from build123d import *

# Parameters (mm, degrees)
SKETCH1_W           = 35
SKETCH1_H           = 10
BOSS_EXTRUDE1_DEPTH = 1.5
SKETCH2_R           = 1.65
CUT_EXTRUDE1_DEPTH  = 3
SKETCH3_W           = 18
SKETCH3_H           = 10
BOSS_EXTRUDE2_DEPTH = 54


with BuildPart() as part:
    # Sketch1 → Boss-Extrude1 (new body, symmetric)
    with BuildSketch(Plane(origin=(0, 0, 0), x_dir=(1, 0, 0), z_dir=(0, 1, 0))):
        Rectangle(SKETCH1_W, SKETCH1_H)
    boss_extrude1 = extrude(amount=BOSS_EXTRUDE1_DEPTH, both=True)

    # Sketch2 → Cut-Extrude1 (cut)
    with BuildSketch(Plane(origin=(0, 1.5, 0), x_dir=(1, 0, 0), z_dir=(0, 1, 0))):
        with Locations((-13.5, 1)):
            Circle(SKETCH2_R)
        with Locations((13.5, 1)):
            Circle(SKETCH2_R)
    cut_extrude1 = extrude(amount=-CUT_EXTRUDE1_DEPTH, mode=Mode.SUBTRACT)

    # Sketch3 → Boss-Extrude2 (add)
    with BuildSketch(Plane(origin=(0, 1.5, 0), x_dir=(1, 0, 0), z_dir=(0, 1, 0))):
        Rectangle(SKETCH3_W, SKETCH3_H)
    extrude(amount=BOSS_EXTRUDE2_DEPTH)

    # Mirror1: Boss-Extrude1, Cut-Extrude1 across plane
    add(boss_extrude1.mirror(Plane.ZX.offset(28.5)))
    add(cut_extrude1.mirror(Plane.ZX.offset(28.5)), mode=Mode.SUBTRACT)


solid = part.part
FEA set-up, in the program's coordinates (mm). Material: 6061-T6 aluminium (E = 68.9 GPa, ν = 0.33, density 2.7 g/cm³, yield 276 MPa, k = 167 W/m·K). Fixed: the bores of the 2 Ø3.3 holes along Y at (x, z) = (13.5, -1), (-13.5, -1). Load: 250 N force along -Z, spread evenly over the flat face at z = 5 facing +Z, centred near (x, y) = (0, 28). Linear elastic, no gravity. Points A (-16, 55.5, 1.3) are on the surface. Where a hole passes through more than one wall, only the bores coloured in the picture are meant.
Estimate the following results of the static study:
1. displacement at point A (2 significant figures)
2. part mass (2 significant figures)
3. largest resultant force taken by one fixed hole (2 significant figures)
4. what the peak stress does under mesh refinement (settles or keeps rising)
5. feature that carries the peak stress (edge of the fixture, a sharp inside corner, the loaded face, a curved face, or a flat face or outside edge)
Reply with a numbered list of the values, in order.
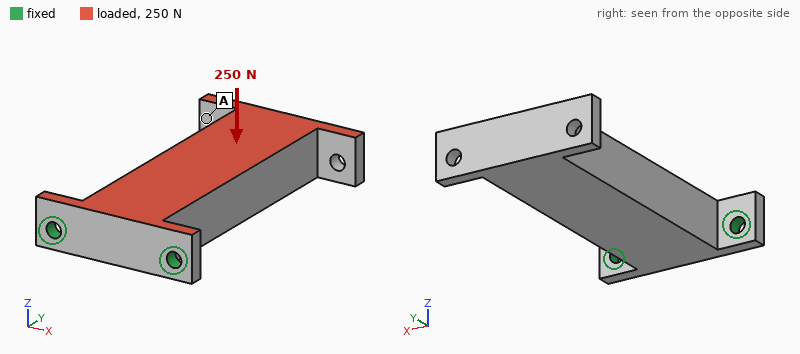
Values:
1. 0.42 mm
2. 32 g
3. 130 N
4. keeps rising
5. edge of the fixture
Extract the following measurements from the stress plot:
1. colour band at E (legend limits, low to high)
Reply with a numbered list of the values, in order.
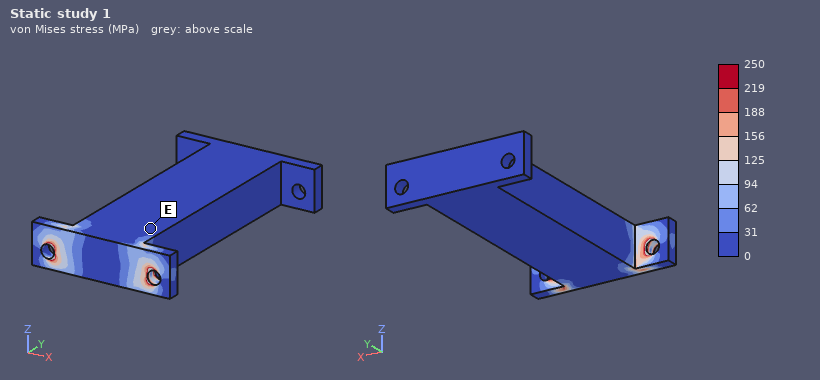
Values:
1. 0 to 31 MPa
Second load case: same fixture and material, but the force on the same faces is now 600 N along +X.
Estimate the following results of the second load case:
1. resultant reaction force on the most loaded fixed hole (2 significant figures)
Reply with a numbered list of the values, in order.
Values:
1. 870 N
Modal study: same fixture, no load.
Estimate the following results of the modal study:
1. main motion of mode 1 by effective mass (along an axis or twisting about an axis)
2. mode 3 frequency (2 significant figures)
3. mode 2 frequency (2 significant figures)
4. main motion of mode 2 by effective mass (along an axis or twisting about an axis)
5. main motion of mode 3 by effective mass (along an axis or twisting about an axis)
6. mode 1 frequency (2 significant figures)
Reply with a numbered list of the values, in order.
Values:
1. along Z
2. 8100 Hz
3. 2400 Hz
4. along X
5. twisting about Y
6. 800 Hz
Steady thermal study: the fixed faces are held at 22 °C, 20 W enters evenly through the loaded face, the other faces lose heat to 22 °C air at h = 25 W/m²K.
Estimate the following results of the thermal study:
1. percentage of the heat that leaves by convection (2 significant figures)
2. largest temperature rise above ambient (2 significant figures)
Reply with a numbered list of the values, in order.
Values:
1. 8.4 %
2. 28 K
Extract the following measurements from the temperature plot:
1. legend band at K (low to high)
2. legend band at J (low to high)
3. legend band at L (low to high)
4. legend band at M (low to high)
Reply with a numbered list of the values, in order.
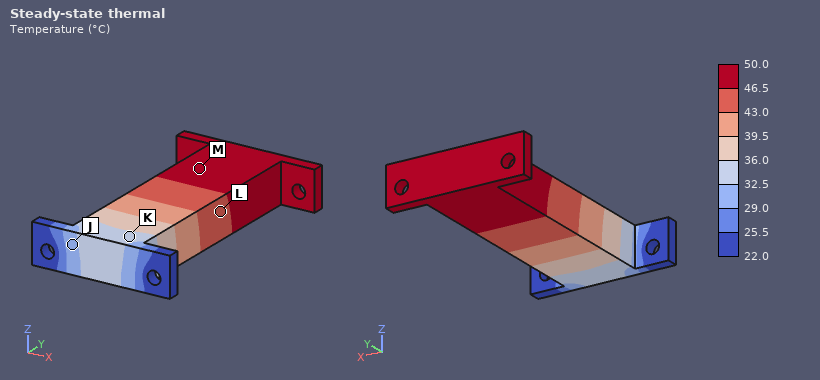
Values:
1. 32.5 to 36.0 °C
2. 29.0 to 32.5 °C
3. 43.0 to 46.5 °C
4. 46.5 to 50.0 °C
